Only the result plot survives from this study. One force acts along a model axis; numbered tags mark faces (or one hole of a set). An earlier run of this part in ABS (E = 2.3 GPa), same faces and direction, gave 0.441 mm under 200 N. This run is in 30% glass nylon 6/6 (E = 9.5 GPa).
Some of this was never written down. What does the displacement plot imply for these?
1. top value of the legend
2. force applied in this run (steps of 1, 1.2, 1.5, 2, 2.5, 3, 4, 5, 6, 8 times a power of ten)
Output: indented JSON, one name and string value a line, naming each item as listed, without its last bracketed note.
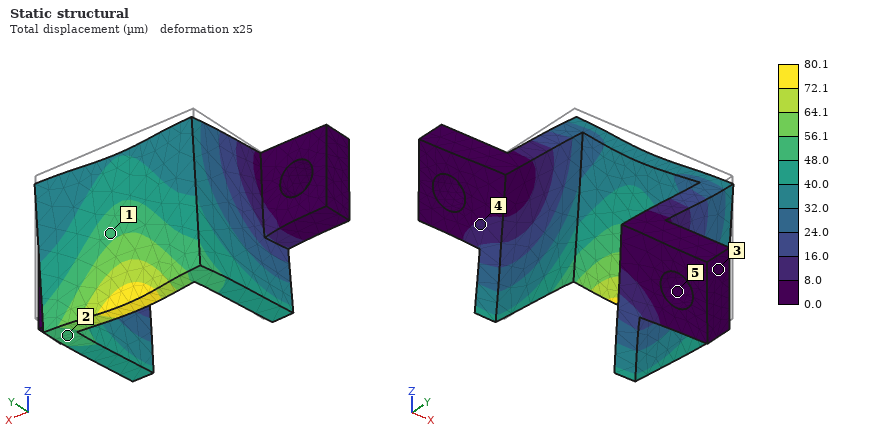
{
  "top value of the legend": "80.1 µm",
  "force applied in this run": "150 N"
}
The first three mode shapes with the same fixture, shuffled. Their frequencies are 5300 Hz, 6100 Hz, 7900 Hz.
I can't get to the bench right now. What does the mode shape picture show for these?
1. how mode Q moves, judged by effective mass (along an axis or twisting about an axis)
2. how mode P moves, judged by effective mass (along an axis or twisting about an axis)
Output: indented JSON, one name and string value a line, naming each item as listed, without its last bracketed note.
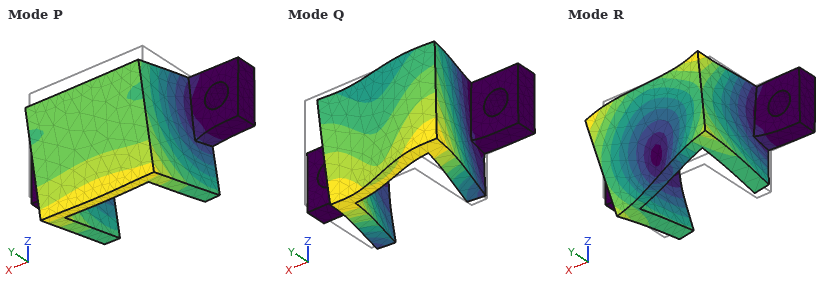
{
  "how mode Q moves, judged by effective mass": "along X",
  "how mode P moves, judged by effective mass": "along Z"
}
